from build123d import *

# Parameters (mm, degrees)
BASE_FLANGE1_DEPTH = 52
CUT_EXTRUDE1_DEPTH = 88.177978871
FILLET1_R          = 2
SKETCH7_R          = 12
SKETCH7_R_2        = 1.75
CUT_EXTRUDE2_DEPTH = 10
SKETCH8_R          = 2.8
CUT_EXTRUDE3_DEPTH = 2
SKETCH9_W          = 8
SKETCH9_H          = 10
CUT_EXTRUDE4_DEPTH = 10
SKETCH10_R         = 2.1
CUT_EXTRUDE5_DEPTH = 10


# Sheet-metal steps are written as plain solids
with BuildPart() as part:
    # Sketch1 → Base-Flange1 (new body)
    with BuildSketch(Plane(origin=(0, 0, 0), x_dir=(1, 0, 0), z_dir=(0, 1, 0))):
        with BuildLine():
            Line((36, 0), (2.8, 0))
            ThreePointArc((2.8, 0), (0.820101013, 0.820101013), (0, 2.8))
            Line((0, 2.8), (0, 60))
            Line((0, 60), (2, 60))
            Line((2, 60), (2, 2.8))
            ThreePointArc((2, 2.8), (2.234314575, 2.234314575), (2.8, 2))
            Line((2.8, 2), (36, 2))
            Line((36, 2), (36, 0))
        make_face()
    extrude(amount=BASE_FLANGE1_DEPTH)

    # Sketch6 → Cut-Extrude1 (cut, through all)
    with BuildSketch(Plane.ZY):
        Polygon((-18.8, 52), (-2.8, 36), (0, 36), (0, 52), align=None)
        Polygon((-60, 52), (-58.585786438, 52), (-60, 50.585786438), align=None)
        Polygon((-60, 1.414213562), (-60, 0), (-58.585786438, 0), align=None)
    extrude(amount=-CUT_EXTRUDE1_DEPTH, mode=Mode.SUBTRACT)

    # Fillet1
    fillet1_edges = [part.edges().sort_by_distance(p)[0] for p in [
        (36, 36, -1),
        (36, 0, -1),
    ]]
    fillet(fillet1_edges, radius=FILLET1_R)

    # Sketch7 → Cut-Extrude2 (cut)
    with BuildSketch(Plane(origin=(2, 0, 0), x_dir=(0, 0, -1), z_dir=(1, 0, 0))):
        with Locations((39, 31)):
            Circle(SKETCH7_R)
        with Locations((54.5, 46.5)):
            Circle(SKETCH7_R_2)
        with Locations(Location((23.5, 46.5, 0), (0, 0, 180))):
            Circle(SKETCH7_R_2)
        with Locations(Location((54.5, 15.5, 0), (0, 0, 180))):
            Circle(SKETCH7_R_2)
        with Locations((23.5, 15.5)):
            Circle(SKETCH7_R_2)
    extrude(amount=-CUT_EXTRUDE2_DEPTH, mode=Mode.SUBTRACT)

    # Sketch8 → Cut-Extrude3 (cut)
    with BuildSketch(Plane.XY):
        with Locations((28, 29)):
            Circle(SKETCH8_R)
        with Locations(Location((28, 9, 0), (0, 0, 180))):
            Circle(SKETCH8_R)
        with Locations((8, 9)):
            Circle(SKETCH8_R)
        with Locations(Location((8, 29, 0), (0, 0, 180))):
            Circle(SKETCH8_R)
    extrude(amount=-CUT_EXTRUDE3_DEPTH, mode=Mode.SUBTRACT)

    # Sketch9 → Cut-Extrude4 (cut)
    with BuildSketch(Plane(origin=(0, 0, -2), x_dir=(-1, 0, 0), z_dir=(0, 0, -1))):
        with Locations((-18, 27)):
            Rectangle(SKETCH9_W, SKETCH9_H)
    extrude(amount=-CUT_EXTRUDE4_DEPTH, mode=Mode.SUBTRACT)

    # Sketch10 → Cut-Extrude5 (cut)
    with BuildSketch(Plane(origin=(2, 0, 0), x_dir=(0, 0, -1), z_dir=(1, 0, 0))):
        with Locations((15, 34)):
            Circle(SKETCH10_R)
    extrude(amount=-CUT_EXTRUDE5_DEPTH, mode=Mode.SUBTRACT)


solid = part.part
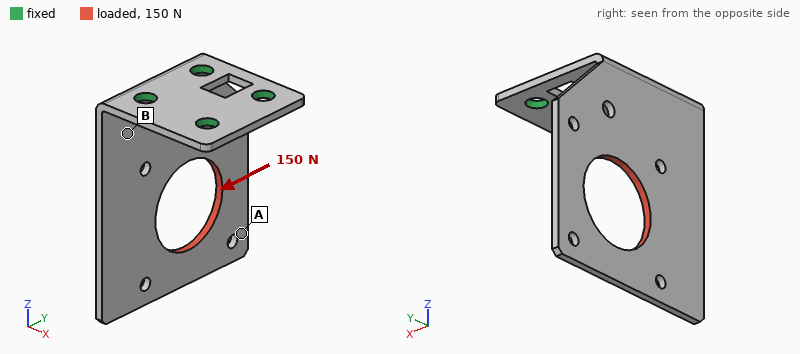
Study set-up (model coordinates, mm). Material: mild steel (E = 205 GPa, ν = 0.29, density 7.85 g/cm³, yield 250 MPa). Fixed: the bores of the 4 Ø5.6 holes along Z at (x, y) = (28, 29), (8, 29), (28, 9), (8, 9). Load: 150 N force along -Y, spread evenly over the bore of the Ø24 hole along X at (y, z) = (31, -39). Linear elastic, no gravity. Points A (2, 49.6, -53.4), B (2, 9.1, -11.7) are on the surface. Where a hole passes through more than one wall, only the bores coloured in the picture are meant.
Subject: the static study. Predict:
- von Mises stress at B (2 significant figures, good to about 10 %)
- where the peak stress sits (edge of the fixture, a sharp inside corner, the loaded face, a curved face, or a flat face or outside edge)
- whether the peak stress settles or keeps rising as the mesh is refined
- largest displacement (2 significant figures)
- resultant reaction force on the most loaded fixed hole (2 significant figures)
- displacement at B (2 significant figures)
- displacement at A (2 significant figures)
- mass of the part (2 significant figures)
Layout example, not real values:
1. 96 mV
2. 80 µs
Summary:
1. 16 MPa
2. edge of the fixture
3. keeps rising
4. 46 µm
5. 270 N
6. 8.9 µm
7. 42 µm
8. 54 g
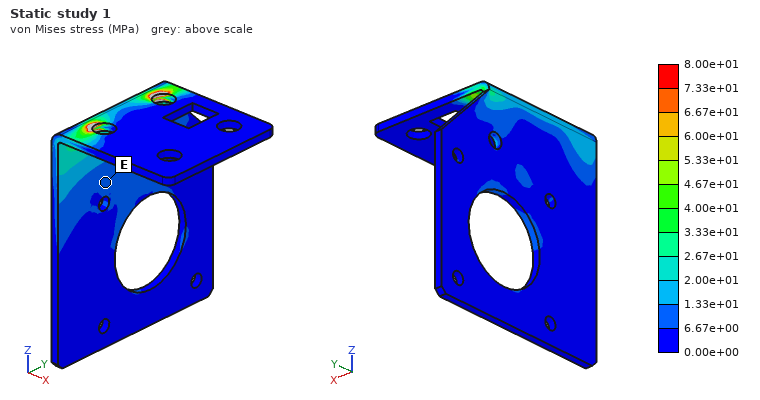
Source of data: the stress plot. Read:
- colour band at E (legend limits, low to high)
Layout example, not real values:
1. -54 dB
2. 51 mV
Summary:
1. 6.67e+00 to 1.33e+01 MPa
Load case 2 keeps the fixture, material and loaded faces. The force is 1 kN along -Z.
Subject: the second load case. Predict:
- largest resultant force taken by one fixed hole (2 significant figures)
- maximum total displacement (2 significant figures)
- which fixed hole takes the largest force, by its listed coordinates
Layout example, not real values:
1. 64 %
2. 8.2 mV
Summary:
1. 1.0 kN
2. 0.25 mm
3. (8, 29)
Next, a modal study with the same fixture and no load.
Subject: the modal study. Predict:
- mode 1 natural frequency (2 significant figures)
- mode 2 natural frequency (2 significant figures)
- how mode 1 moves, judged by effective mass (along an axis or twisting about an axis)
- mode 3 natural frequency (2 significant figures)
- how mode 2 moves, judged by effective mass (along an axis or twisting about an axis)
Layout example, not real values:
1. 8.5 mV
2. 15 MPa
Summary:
1. 400 Hz
2. 1000 Hz
3. along X
4. 2200 Hz
5. twisting about Z
